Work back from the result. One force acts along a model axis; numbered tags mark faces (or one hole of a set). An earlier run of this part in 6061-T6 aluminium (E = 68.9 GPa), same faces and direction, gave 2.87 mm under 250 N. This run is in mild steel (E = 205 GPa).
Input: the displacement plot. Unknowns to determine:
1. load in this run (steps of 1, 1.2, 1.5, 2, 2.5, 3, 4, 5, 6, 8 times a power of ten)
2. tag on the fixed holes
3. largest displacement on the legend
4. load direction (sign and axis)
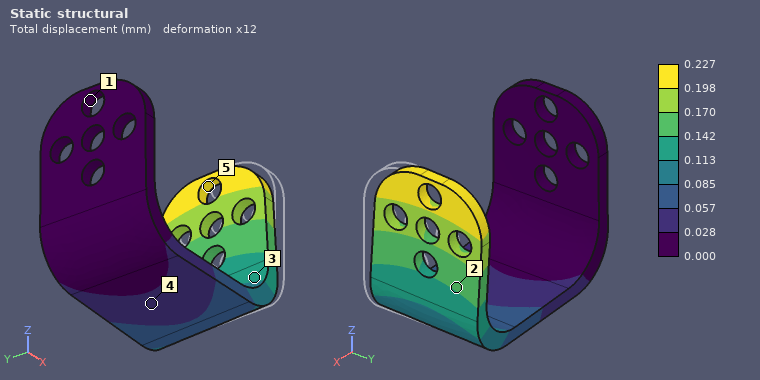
60 N
1
0.227 mm
+Y
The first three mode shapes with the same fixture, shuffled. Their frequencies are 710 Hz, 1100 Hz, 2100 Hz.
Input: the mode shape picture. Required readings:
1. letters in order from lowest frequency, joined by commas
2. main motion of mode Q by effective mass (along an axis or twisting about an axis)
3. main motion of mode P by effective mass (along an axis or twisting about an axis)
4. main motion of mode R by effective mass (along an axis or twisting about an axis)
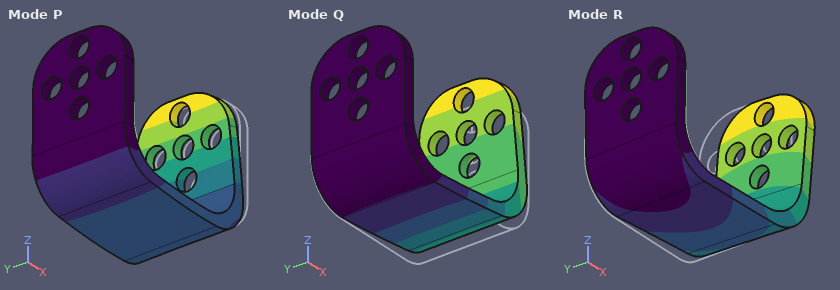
Q, R, P
along Z
along X
along Y
